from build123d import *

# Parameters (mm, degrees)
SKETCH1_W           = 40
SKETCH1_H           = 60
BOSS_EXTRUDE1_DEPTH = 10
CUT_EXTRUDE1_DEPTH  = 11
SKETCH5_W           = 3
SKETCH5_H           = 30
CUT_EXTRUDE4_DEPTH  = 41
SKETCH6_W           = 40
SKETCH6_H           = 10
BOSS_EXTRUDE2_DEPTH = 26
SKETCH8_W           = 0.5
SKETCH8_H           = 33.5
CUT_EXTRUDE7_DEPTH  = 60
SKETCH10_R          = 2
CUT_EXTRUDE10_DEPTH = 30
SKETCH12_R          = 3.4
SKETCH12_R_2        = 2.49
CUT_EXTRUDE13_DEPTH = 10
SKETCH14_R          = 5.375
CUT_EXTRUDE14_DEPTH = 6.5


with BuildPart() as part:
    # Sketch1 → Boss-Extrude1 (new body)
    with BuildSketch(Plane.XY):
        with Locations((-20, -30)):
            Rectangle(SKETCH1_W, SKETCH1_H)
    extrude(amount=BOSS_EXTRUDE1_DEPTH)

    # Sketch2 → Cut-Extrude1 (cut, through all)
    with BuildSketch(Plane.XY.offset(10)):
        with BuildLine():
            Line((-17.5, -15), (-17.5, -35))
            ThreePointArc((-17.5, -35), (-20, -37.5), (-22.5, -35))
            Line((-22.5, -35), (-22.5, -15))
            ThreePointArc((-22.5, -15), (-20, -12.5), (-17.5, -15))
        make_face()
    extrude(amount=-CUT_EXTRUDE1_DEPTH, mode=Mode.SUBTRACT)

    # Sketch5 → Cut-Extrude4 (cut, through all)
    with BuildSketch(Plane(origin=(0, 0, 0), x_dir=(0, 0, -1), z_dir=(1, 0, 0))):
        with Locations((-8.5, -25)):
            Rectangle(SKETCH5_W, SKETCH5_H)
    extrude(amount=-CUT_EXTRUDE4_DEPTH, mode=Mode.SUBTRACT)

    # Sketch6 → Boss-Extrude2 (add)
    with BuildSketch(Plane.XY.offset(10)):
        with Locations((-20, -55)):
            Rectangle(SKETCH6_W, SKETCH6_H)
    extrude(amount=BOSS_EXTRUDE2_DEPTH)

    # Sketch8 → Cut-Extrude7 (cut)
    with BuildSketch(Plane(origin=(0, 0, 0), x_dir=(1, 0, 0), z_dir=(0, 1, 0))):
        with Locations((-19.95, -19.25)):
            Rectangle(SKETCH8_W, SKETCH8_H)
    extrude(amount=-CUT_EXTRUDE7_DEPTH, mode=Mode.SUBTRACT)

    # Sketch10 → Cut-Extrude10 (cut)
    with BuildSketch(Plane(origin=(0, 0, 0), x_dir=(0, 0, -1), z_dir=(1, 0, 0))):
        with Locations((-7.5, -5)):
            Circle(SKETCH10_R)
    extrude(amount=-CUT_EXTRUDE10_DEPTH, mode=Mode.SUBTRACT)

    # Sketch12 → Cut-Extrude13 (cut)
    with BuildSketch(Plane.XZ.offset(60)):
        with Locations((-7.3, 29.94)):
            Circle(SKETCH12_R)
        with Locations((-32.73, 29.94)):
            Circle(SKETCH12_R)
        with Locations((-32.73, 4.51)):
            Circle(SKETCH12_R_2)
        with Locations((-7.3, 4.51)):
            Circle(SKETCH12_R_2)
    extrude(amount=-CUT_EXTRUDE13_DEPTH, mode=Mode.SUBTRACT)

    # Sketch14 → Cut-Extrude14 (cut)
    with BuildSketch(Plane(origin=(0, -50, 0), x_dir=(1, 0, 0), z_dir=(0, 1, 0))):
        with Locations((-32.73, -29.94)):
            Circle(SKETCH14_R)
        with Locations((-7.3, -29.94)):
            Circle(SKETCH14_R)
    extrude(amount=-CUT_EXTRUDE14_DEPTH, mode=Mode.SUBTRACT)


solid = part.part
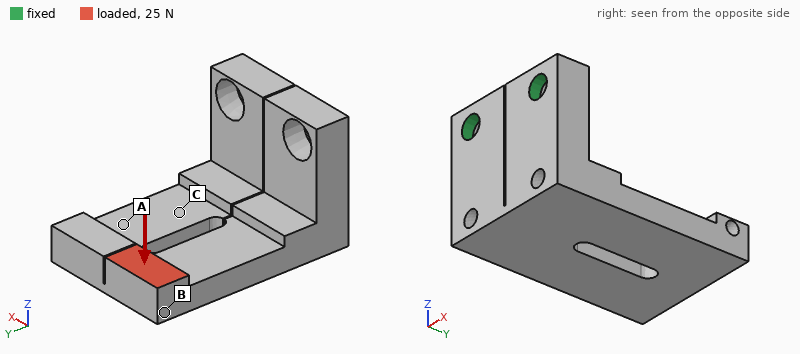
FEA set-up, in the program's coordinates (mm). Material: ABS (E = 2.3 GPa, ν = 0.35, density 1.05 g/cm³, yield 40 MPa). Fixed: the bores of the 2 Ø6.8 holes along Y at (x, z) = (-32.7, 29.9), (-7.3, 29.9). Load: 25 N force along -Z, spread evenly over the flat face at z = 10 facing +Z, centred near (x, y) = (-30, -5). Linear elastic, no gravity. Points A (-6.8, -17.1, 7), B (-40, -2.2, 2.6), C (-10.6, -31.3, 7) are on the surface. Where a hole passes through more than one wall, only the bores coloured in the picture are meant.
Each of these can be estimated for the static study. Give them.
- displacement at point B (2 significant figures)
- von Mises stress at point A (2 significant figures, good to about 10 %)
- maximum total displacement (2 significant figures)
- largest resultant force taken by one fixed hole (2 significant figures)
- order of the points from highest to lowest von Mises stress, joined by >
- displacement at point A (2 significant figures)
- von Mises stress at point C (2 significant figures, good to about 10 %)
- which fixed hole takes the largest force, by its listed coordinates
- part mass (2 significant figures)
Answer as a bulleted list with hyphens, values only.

- 0.80 mm
- 1.3 MPa
- 0.85 mm
- 20 N
- C > A > B
- 0.45 mm
- 2.2 MPa
- (-32.7, 29.9)
- 29 g
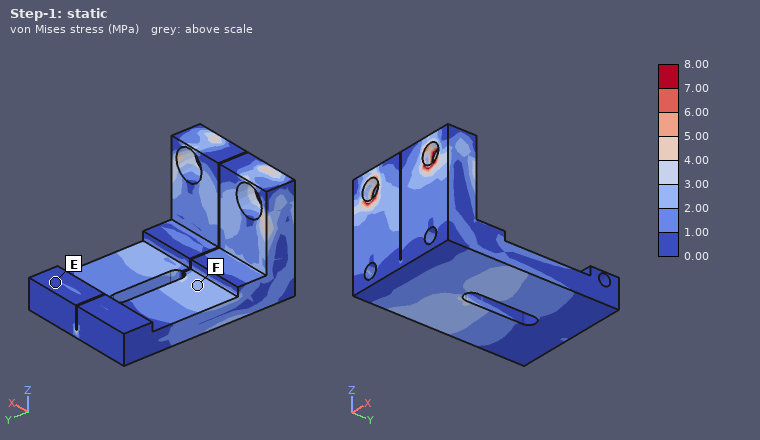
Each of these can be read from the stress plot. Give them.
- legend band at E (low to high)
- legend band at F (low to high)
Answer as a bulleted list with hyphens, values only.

- 0.00 to 1.00 MPa
- 2.00 to 3.00 MPa
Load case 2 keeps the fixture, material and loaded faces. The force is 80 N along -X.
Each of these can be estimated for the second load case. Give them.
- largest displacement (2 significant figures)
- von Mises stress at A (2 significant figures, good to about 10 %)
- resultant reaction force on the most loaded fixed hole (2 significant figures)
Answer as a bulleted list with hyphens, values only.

- 0.94 mm
- 1.4 MPa
- 120 N
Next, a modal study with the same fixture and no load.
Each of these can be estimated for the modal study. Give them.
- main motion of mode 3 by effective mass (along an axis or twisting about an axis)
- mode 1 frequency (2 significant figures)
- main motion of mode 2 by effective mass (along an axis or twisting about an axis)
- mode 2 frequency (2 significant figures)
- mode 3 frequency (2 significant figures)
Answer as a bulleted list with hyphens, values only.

- along Y
- 350 Hz
- along X
- 630 Hz
- 1100 Hz
